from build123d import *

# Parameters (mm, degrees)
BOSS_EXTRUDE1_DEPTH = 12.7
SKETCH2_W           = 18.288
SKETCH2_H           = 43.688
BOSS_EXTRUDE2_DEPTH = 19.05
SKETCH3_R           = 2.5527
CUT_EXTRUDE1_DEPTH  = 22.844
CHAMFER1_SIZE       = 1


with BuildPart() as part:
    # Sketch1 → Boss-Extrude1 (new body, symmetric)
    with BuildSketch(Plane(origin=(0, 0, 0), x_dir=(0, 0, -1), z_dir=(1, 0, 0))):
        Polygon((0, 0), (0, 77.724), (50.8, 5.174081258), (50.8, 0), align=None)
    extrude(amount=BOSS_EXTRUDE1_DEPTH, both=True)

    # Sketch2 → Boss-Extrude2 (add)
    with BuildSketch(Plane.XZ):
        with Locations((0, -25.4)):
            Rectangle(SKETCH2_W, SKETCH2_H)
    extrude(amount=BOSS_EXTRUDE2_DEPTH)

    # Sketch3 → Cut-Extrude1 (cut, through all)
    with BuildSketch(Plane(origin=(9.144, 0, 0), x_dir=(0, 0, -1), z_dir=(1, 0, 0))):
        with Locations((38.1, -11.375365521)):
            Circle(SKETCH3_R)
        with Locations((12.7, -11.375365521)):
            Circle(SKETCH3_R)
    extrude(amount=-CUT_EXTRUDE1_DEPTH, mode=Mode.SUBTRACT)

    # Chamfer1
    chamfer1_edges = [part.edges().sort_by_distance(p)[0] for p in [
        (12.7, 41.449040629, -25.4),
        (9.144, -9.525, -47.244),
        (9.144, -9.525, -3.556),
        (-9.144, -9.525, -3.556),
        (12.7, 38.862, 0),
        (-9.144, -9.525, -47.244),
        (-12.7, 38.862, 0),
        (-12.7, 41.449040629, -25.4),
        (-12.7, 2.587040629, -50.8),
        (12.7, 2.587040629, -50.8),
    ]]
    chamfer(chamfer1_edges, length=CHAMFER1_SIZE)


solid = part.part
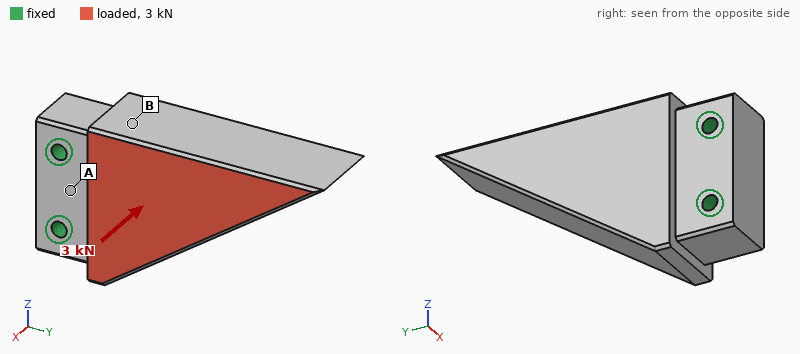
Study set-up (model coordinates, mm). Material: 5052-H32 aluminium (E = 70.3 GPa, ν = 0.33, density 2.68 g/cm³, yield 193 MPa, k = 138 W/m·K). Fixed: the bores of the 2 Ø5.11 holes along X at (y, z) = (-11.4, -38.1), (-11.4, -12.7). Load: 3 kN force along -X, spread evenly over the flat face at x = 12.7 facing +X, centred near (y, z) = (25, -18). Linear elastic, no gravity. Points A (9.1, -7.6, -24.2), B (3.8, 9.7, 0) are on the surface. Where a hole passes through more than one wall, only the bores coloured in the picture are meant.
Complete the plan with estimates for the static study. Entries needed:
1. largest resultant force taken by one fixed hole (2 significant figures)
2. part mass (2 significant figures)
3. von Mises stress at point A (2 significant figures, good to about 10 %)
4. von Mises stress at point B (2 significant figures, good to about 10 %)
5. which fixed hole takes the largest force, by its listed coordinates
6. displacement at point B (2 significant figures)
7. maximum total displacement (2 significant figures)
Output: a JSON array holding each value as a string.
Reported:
["2.0 kN", "180 g", "18 MPa", "8.3 MPa", "(-11.4, -12.7)", "0.021 mm", "0.11 mm"]
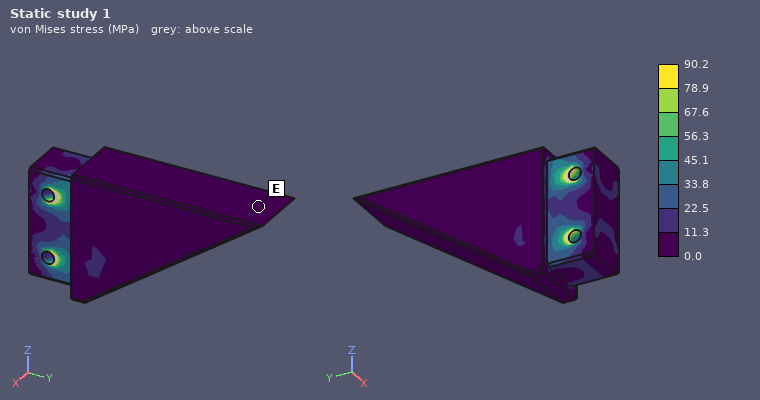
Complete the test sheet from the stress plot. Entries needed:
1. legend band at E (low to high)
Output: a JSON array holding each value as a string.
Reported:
["0.0 to 11.3 MPa"]
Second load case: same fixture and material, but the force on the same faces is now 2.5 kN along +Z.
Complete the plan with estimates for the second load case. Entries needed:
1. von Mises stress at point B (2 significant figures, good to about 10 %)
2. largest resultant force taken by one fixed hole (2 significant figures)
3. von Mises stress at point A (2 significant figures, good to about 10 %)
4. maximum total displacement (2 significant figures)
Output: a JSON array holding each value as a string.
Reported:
["5.6 MPa", "3.5 kN", "11 MPa", "33 µm"]
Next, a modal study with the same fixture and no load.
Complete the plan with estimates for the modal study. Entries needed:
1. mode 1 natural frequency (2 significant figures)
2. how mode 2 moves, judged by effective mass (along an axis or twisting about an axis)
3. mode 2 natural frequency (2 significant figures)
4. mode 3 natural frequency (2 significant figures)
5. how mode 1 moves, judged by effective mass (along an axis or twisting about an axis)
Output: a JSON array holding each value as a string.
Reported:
["3000 Hz", "along Z", "5400 Hz", "11 kHz", "along X"]
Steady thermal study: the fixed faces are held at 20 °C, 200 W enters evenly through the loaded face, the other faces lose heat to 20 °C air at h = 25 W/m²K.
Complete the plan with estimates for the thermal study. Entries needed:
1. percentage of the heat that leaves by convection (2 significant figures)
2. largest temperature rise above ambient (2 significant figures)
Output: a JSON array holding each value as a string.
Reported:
["4.2 %", "67 K"]
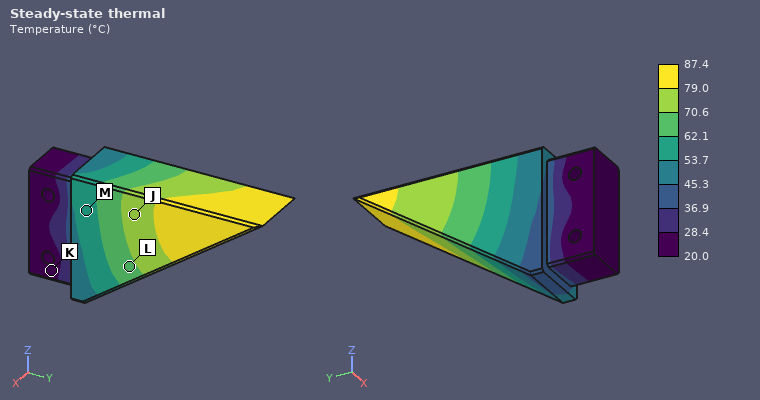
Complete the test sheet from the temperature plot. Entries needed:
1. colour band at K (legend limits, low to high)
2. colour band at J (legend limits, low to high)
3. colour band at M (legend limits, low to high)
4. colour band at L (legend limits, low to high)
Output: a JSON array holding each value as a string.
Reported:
["20.0 to 28.4 °C", "70.6 to 79.0 °C", "53.7 to 62.1 °C", "62.1 to 70.6 °C"]
